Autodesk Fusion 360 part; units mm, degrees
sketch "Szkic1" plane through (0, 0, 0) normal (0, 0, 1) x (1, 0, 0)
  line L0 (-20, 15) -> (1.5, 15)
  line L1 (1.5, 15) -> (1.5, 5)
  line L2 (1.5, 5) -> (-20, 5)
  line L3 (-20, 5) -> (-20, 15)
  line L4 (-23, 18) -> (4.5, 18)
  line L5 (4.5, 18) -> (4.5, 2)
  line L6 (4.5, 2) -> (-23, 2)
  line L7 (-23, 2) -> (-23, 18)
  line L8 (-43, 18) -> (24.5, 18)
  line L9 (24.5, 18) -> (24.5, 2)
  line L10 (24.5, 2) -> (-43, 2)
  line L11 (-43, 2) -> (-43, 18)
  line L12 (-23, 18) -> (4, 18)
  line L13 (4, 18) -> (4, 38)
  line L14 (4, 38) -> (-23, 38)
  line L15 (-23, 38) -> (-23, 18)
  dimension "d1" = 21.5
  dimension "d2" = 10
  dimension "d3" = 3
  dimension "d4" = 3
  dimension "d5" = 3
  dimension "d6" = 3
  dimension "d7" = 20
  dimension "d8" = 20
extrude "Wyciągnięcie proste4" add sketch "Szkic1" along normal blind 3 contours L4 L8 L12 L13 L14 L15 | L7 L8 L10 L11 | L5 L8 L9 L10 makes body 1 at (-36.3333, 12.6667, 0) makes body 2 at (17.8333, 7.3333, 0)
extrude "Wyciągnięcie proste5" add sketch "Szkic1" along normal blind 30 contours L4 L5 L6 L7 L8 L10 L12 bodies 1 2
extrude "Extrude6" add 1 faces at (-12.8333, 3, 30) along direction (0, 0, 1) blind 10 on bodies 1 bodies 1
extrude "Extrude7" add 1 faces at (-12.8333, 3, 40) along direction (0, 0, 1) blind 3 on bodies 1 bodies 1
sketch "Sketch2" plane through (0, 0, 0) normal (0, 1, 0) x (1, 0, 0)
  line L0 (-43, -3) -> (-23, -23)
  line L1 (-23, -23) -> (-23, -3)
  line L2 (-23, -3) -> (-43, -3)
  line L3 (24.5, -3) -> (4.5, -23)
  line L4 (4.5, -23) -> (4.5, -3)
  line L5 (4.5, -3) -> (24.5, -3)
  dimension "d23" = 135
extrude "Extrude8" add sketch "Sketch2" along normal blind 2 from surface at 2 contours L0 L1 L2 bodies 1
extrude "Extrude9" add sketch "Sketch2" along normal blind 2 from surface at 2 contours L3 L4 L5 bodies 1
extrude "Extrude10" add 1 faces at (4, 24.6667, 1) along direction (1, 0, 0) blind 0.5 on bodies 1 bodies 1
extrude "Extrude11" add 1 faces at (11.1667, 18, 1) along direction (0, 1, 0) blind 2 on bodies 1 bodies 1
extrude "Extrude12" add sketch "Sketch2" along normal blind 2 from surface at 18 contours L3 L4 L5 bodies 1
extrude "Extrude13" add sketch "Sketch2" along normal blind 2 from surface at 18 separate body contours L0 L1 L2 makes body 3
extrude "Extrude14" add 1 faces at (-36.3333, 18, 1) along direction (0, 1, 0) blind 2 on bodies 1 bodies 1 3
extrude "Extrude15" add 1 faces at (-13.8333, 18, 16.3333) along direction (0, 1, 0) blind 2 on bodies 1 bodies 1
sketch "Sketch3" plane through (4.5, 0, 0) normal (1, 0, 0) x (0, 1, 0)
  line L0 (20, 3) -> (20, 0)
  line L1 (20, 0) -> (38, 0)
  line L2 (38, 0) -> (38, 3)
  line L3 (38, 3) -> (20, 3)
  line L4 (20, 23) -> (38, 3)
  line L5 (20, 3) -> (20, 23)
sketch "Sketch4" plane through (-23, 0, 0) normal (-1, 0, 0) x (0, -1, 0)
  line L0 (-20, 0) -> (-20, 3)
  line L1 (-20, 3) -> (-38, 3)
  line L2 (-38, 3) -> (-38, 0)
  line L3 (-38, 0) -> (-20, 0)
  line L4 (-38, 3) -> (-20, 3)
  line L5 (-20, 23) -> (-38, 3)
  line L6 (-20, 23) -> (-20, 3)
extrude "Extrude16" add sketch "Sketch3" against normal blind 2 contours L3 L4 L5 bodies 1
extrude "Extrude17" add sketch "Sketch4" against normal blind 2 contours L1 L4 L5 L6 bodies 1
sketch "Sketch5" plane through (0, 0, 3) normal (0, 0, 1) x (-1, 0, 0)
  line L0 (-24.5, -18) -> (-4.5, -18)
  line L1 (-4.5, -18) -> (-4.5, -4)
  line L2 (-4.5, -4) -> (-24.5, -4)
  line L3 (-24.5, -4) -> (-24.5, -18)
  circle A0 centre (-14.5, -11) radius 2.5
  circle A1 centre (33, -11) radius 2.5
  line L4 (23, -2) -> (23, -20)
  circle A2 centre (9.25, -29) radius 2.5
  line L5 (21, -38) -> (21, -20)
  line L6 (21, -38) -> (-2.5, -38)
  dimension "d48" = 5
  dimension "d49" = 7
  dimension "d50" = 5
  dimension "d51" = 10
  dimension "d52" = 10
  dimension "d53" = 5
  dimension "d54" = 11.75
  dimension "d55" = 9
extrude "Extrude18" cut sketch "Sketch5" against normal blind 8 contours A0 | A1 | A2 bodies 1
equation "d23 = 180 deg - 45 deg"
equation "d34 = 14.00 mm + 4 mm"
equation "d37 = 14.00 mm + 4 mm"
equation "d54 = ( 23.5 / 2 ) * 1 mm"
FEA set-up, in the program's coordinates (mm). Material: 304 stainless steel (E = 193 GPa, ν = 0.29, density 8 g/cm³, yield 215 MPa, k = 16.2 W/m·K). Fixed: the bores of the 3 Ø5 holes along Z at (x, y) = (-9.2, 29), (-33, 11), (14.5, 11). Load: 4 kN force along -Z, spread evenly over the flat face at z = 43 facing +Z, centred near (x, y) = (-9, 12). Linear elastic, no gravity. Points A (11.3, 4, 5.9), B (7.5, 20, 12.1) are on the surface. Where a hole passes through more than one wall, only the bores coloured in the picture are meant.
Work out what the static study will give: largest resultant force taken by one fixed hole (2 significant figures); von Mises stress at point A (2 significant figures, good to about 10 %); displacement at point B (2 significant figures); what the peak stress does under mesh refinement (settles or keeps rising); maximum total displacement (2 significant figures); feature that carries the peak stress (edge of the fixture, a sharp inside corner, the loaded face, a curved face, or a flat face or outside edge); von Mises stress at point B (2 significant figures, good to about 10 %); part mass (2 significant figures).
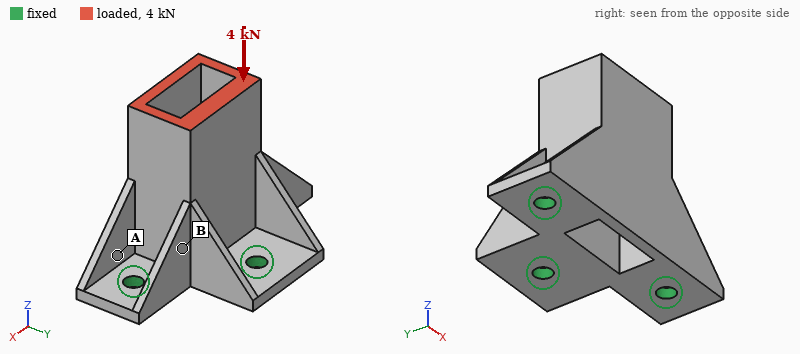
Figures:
2.0 kN
72 MPa
7.7 µm
keeps rising
26 µm
edge of the fixture
32 MPa
140 g
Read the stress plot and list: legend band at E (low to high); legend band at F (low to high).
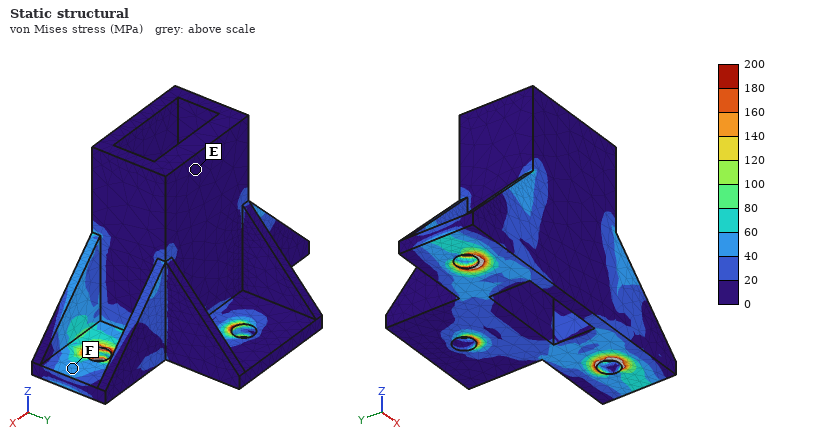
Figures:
0 to 20 MPa
40 to 60 MPa
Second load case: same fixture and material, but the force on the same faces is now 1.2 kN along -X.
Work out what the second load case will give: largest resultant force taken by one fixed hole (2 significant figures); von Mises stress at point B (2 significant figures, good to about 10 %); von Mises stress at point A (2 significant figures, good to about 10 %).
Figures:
1.2 kN
26 MPa
41 MPa
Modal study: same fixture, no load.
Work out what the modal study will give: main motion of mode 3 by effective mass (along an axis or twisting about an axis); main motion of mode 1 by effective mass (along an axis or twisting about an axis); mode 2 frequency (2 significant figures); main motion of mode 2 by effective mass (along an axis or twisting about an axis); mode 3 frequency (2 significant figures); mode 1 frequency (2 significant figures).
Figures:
along Z
along Y
7100 Hz
along X
9200 Hz
3300 Hz
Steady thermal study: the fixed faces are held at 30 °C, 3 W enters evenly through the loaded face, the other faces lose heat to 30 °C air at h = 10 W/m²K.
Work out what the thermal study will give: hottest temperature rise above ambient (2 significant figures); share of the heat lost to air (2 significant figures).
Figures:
25 K
36 %
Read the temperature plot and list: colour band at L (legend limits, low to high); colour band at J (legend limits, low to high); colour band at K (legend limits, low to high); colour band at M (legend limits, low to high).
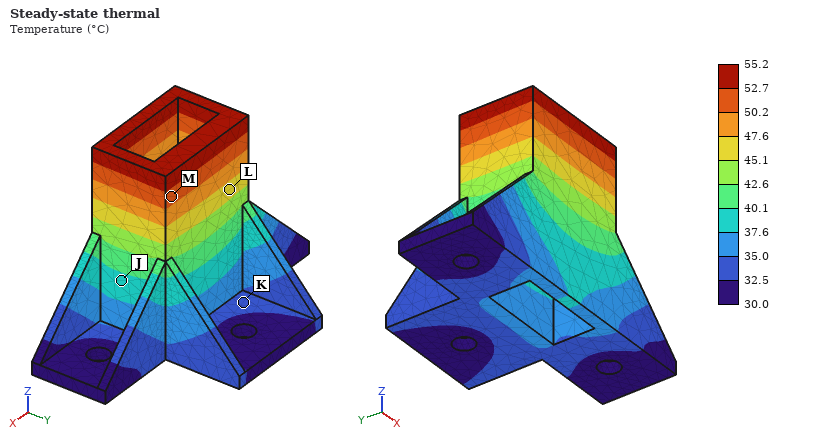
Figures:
45.1 to 47.6 °C
37.6 to 40.1 °C
32.5 to 35.0 °C
50.2 to 52.7 °C
